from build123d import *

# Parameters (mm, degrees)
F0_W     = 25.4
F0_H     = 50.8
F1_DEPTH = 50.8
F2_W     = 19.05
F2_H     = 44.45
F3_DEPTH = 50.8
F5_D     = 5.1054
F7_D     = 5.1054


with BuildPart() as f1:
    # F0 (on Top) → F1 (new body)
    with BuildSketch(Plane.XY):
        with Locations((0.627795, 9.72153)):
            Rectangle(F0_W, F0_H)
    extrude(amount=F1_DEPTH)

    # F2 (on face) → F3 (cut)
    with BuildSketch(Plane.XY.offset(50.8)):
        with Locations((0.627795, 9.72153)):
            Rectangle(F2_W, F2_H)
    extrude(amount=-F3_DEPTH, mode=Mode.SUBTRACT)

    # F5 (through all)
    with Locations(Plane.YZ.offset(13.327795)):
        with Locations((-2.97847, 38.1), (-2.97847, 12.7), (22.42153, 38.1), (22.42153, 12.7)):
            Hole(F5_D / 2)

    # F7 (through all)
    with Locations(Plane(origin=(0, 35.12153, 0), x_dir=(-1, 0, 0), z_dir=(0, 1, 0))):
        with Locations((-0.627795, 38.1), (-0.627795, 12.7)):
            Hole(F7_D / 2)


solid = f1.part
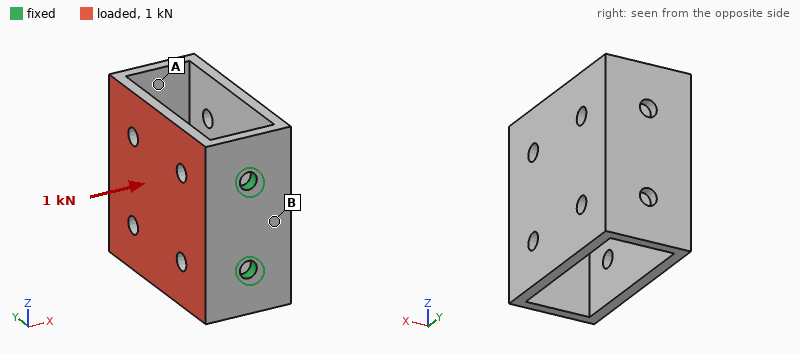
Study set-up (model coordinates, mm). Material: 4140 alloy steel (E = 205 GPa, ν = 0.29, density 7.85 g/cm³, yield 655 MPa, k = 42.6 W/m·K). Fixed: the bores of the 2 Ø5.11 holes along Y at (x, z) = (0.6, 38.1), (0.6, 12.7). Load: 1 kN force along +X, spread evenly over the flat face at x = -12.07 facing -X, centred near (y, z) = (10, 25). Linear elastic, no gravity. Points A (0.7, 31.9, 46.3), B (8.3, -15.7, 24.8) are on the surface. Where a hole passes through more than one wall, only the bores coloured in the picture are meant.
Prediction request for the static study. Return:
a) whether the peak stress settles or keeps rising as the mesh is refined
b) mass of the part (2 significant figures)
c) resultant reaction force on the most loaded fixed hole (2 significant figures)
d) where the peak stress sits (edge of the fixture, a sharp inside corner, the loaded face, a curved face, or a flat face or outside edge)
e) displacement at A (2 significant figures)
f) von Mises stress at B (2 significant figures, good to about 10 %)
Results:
keeps rising
170 g
500 N
edge of the fixture
0.22 mm
73 MPa
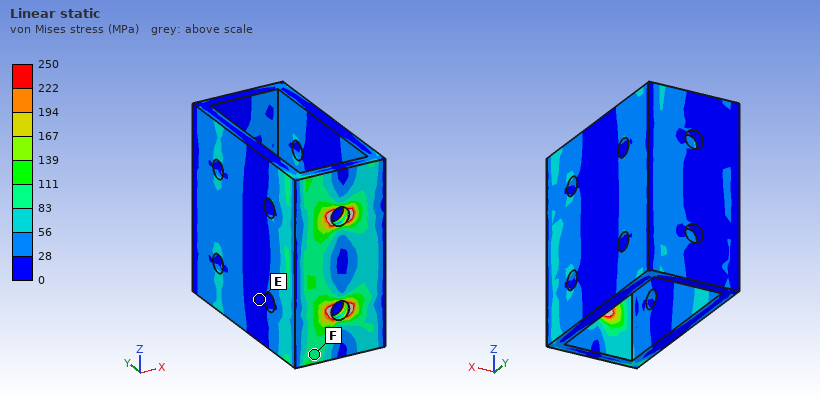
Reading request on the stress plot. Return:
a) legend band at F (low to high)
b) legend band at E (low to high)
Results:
83 to 111 MPa
0 to 28 MPa
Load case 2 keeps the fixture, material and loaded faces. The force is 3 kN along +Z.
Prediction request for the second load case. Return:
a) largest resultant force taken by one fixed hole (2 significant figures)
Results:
3.1 kN
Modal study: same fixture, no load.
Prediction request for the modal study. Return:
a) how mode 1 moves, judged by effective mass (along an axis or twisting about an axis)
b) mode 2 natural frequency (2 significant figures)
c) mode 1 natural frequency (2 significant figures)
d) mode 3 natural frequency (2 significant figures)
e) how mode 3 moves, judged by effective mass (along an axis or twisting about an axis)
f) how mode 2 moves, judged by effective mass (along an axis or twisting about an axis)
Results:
along X
2500 Hz
890 Hz
3000 Hz
twisting about Y
along Z
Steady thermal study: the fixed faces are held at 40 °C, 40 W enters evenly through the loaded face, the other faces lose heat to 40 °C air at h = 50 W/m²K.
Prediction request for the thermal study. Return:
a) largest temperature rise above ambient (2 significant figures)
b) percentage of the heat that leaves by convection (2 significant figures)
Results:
74 K
51 %
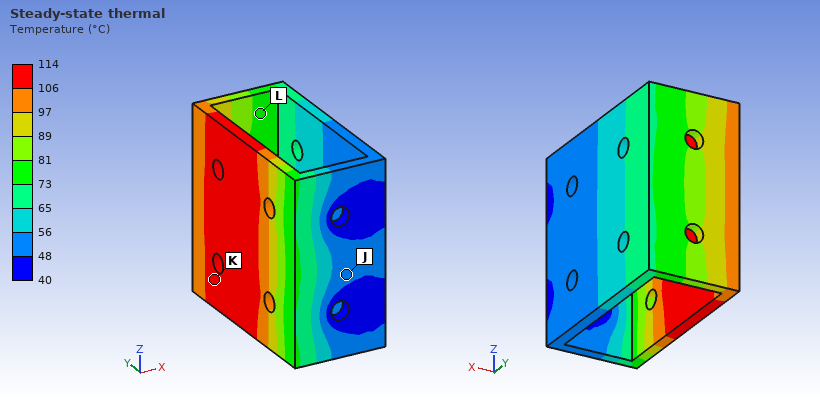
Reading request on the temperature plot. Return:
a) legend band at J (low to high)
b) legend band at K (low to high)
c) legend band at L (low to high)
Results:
48 to 56 °C
106 to 114 °C
73 to 81 °C
